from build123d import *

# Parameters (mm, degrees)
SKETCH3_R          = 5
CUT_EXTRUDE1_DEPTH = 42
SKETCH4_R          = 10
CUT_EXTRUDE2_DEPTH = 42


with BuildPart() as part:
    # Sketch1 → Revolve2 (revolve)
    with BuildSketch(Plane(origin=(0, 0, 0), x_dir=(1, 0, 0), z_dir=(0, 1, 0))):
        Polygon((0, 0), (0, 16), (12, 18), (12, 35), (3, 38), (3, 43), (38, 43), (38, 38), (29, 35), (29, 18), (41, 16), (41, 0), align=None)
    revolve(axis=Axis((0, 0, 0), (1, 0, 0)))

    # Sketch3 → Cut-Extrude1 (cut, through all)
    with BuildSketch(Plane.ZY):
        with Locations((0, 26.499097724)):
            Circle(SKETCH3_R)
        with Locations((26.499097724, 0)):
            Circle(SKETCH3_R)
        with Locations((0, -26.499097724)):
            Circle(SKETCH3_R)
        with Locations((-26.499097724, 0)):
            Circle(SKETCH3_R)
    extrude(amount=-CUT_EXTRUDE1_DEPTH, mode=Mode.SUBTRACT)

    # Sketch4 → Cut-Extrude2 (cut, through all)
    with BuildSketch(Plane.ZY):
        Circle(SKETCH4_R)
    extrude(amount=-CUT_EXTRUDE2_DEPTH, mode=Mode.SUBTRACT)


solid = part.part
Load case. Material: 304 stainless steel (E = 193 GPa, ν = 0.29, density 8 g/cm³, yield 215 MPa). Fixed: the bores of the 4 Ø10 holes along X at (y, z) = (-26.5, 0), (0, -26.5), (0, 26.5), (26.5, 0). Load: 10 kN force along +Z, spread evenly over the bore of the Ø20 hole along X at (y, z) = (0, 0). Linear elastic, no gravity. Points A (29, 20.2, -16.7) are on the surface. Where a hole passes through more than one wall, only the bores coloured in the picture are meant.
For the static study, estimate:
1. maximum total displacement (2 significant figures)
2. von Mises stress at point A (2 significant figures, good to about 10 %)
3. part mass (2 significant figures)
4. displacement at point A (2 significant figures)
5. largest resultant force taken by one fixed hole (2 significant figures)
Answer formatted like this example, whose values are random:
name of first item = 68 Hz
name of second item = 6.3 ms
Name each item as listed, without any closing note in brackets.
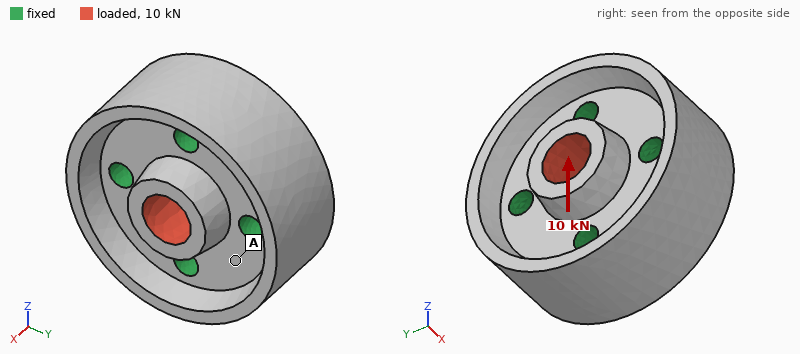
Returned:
maximum total displacement = 1.8 µm
von Mises stress at point A = 2.2 MPa
part mass = 1.1 kg
displacement at point A = 0.27 µm
largest resultant force taken by one fixed hole = 3.1 kN
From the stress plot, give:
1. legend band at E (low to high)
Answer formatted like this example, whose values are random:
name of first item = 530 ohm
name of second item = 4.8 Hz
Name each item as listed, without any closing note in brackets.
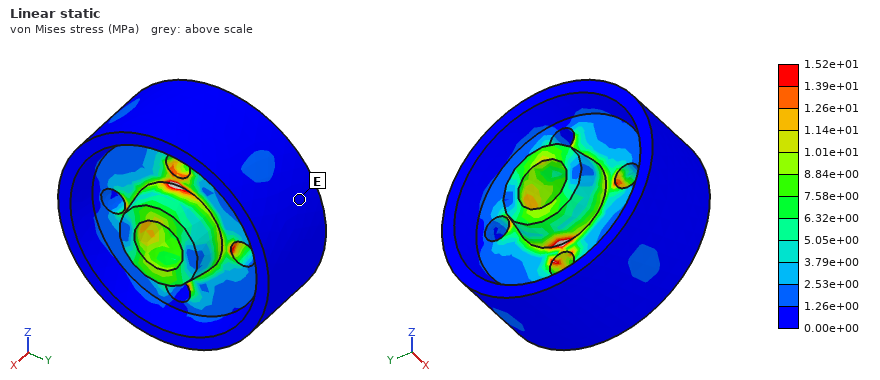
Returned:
legend band at E = 0.00e+00 to 1.26e+00 MPa
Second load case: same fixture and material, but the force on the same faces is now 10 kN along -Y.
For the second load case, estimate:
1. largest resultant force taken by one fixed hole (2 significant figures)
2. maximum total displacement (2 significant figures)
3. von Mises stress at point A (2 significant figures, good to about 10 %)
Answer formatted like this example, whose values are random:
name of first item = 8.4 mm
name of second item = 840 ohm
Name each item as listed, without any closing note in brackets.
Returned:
largest resultant force taken by one fixed hole = 3.1 kN
maximum total displacement = 1.7 µm
von Mises stress at point A = 2.3 MPa
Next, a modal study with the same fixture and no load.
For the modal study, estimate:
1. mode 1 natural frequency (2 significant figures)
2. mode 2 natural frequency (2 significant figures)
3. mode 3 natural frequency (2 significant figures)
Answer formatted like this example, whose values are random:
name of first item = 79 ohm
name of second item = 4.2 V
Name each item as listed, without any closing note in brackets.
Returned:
mode 1 natural frequency = 15 kHz
mode 2 natural frequency = 17 kHz
mode 3 natural frequency = 17 kHz
